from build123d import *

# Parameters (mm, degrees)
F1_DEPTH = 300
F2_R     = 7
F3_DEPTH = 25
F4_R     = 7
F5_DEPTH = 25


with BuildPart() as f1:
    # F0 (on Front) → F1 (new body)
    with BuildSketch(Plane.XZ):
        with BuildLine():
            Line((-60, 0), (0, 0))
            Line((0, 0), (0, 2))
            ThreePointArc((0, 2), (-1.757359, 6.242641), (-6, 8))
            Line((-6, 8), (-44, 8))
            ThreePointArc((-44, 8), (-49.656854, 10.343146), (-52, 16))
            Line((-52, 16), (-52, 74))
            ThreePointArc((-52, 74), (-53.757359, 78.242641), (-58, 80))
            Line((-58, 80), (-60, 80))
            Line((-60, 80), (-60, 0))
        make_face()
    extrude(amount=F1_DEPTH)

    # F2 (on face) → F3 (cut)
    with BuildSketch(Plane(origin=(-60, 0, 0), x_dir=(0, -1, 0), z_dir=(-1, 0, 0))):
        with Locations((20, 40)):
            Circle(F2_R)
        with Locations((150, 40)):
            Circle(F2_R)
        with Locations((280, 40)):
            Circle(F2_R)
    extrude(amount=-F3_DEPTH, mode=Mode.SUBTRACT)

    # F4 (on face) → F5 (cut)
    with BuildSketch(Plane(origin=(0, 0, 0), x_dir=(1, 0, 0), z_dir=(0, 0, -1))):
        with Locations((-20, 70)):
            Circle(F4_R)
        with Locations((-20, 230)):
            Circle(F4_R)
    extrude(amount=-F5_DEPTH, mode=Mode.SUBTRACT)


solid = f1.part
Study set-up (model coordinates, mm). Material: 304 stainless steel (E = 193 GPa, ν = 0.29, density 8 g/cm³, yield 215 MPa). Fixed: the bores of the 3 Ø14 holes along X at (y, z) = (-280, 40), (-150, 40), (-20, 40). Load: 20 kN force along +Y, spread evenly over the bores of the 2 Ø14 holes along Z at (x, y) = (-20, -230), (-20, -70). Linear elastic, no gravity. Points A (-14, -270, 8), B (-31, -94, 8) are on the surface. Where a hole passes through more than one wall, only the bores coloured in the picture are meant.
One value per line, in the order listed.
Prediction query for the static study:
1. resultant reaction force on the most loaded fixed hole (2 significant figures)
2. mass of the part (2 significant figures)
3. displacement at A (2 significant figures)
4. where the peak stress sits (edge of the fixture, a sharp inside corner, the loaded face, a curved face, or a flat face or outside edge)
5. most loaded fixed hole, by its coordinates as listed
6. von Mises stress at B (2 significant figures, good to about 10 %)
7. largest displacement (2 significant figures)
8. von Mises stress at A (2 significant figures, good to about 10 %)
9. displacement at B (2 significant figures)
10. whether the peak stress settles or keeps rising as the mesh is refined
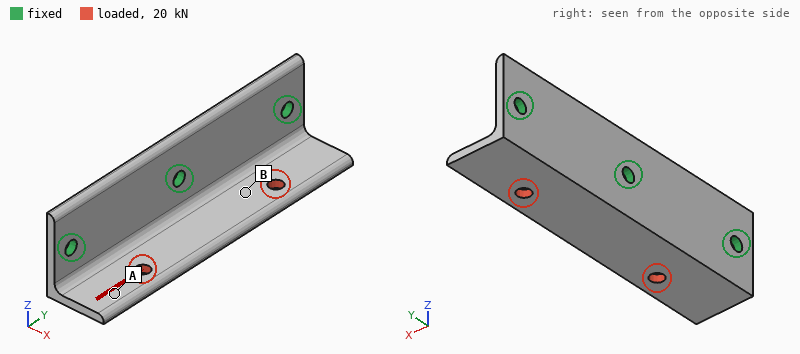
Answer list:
9.0 kN
2.5 kg
0.085 mm
edge of the fixture
(-150, 40)
32 MPa
0.13 mm
15 MPa
0.031 mm
keeps rising
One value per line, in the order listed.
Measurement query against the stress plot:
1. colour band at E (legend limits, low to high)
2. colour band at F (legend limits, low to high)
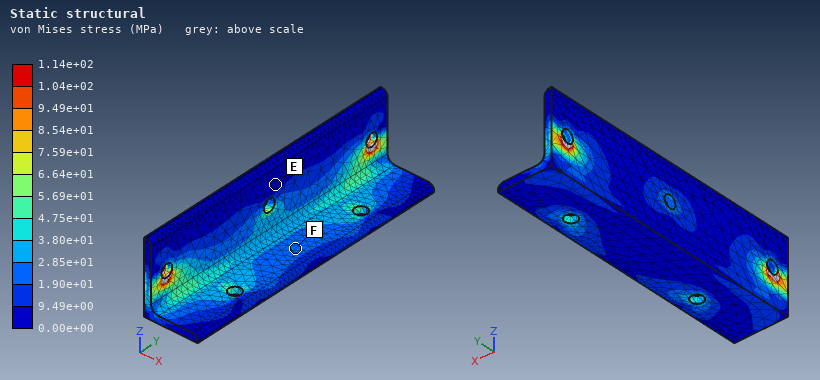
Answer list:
0.00e+00 to 9.49e+00 MPa
1.90e+01 to 2.85e+01 MPa
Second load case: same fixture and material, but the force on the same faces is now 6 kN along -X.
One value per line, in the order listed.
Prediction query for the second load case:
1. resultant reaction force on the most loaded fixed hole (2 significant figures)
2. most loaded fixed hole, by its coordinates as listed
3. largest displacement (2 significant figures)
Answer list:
2.5 kN
(-150, 40)
0.11 mm
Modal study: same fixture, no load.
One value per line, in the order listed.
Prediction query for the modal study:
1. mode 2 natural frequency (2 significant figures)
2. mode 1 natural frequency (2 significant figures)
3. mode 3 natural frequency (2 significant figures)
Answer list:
1300 Hz
1000 Hz
2400 Hz
